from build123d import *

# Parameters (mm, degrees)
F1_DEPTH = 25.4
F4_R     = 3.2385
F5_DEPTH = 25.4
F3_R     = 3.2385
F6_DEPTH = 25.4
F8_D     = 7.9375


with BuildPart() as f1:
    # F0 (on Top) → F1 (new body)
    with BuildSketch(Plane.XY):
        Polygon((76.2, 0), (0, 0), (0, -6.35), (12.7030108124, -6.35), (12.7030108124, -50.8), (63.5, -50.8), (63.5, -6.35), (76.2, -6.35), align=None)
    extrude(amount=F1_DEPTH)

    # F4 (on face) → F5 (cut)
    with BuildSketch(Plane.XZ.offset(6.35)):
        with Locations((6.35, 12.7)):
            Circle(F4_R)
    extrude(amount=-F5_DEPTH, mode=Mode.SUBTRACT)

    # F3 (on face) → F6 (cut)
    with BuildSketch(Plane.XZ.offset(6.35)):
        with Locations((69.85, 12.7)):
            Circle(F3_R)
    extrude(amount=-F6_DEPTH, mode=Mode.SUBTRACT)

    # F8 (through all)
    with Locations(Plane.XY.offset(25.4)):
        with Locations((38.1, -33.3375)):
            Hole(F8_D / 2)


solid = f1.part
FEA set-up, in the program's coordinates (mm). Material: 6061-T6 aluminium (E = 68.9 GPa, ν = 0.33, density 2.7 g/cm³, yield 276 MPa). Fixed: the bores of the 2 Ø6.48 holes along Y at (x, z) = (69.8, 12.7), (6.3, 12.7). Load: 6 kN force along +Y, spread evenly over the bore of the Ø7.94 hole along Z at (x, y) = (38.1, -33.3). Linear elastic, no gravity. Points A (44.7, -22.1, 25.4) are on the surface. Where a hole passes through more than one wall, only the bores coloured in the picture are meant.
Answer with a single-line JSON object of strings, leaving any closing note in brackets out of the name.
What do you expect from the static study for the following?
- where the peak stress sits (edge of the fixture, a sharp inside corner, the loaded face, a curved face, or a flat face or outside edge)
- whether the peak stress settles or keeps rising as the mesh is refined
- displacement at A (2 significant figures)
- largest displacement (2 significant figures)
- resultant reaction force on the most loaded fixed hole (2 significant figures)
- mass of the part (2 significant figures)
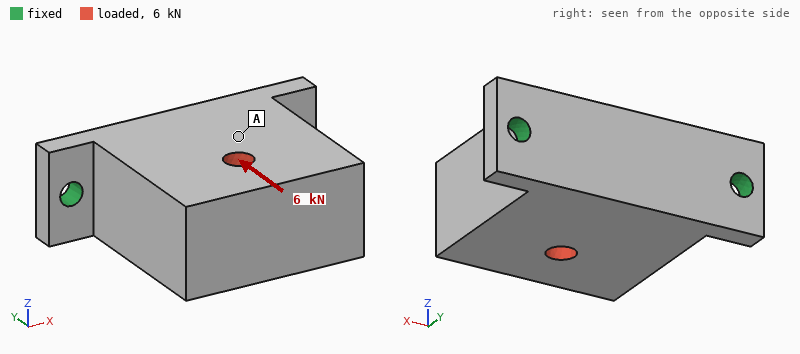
{"where the peak stress sits": "edge of the fixture", "whether the peak stress settles or keeps rising as the mesh is refined": "keeps rising", "displacement at A": "17 µm", "largest displacement": "19 µm", "resultant reaction force on the most loaded fixed hole": "3.3 kN", "mass of the part": "180 g"}
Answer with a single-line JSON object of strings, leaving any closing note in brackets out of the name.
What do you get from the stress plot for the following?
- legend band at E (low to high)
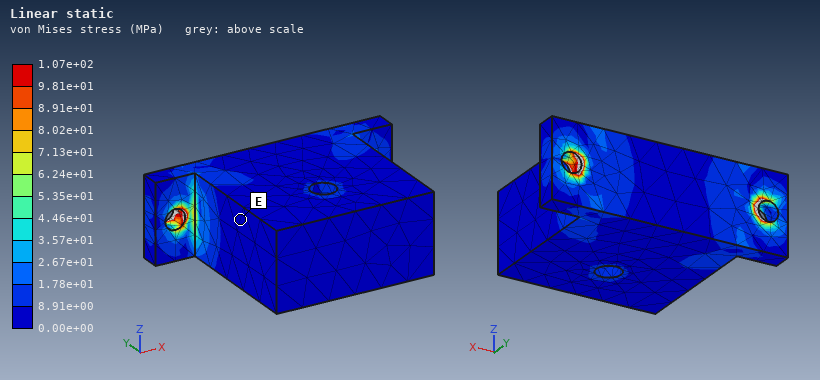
{"legend band at E": "0.00e+00 to 8.91e+00 MPa"}
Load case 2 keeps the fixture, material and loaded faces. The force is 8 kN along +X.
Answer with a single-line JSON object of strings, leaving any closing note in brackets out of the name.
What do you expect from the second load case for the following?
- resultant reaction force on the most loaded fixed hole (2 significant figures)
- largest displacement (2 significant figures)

{"resultant reaction force on the most loaded fixed hole": "5.9 kN", "largest displacement": "51 µm"}
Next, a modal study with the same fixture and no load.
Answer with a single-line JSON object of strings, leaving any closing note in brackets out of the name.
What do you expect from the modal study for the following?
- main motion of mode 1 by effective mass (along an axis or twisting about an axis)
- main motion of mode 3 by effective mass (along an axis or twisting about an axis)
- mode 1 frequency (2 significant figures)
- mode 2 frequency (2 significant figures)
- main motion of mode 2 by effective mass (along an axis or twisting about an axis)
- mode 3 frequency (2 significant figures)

{"main motion of mode 1 by effective mass": "along Z", "main motion of mode 3 by effective mass": "along Y", "mode 1 frequency": "1700 Hz", "mode 2 frequency": "6400 Hz", "main motion of mode 2 by effective mass": "along X", "mode 3 frequency": "7400 Hz"}
